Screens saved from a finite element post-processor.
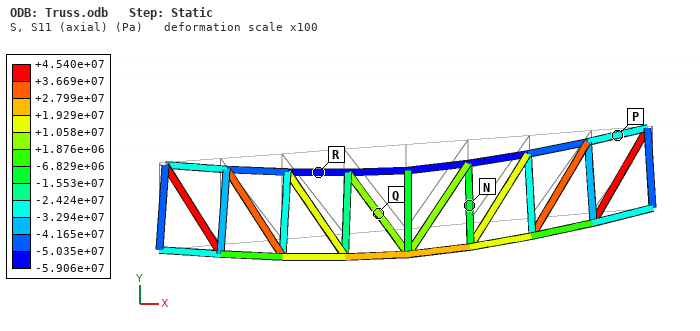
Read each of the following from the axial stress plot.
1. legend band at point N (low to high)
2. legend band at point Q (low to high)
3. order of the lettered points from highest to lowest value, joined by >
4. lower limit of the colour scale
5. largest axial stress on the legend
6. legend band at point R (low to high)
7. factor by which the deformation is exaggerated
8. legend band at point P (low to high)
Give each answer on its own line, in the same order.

-1.553e+07 to -6.829e+06 Pa
+1.876e+06 to +1.058e+07 Pa
Q > N > P > R
-5.906e+07 Pa
+4.540e+07 Pa
-5.906e+07 to -5.035e+07 Pa
100
-3.294e+07 to -2.424e+07 Pa
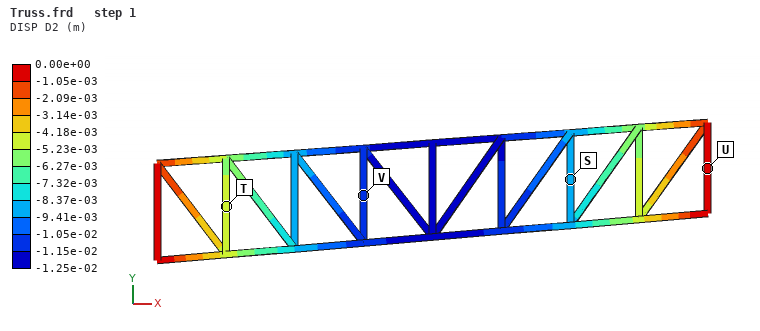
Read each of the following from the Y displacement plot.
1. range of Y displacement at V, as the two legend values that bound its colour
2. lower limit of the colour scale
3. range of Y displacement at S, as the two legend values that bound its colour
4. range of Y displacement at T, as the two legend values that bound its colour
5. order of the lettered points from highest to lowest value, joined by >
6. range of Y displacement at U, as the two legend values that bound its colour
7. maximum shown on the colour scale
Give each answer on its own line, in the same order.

-1.15e-02 to -1.05e-02 m
-1.25e-02 m
-9.41e-03 to -8.37e-03 m
-5.23e-03 to -4.18e-03 m
U > T > S > V
-1.05e-03 to 0.00e+00 m
0.00e+00 m
